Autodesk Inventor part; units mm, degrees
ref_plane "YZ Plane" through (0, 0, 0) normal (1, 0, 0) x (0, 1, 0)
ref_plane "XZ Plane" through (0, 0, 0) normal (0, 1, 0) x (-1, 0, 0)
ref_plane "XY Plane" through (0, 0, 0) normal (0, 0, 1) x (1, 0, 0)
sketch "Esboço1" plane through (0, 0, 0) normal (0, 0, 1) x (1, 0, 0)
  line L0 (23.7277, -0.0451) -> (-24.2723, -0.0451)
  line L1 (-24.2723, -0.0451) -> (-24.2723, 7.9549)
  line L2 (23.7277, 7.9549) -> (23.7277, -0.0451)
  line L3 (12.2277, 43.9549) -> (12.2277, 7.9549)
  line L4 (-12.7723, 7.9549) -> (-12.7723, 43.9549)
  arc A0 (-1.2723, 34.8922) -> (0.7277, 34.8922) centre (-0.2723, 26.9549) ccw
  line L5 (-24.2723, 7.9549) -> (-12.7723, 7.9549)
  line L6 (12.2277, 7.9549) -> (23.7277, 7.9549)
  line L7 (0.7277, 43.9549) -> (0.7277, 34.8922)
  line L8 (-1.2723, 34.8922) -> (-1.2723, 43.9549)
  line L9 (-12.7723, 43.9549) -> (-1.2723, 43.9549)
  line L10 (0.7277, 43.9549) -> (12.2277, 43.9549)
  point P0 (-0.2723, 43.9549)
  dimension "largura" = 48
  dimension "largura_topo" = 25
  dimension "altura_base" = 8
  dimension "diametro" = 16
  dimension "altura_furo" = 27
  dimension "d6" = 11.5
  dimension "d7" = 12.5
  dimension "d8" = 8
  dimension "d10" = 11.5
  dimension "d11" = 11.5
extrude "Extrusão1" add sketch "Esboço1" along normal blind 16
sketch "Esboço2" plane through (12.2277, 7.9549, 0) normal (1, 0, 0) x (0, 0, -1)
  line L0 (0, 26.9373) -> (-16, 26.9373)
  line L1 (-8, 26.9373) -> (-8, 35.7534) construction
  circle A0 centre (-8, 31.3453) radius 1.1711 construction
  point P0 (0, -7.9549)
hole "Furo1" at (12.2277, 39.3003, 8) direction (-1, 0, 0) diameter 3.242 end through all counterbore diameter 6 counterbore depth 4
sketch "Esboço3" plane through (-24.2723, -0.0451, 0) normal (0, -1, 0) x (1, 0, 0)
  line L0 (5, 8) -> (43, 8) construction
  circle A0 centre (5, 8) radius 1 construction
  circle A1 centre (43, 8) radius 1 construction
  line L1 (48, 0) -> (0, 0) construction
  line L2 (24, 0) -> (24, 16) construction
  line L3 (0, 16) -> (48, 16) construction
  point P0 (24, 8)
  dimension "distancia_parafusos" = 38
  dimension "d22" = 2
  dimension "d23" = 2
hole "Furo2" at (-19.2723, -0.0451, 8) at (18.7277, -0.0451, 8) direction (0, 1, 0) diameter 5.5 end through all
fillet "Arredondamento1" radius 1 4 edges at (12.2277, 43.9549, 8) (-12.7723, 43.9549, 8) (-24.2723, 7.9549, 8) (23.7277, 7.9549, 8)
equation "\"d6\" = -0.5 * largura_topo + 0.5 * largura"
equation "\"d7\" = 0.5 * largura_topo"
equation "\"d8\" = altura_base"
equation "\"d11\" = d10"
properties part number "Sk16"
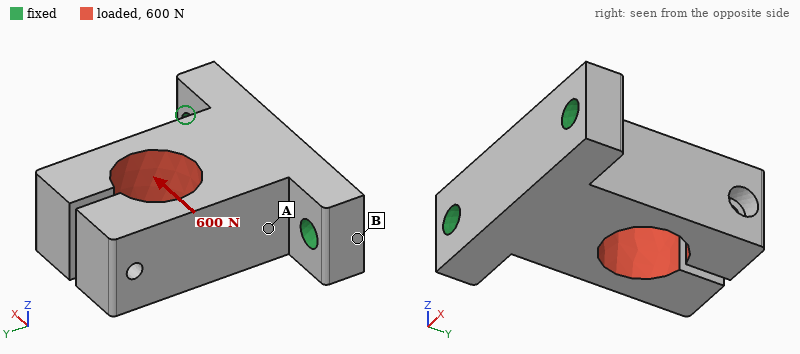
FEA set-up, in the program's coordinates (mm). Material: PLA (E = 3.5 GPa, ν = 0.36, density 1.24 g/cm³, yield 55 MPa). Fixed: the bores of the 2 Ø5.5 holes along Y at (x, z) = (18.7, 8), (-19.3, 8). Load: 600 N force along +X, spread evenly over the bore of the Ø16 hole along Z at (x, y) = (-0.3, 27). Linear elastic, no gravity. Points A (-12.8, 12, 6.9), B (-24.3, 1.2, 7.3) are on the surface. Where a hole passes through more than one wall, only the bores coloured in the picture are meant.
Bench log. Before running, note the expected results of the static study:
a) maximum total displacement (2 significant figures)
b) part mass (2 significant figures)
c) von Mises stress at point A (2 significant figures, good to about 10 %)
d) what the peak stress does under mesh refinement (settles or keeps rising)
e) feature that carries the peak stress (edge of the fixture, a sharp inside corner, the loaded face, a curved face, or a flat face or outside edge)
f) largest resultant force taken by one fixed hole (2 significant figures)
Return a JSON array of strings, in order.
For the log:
["0.61 mm", "20 g", "9.3 MPa", "keeps rising", "edge of the fixture", "530 N"]
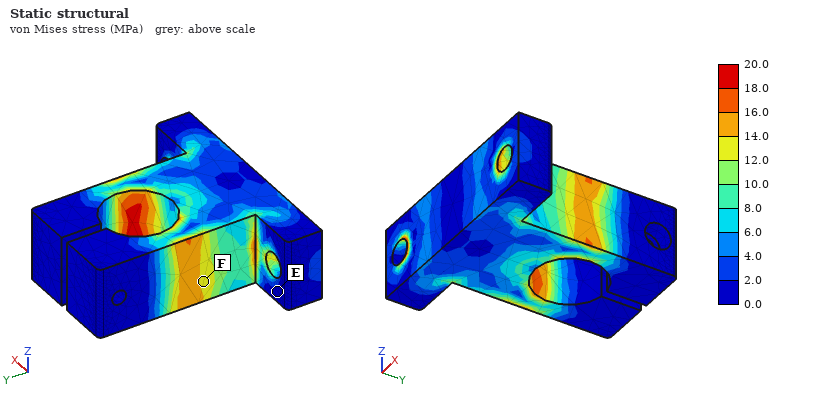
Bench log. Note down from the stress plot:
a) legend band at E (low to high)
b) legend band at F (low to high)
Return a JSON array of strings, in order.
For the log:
["0.0 to 2.0 MPa", "12.0 to 14.0 MPa"]
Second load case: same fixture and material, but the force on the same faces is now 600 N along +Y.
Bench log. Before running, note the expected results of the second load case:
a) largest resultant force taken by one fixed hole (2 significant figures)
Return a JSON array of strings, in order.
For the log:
["320 N"]
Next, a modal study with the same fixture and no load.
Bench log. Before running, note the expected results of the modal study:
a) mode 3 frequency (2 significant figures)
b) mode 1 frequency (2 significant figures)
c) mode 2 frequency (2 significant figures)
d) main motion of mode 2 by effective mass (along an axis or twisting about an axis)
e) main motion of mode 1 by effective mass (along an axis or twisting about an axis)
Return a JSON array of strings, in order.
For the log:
["1500 Hz", "1300 Hz", "1400 Hz", "along X", "along Z"]
